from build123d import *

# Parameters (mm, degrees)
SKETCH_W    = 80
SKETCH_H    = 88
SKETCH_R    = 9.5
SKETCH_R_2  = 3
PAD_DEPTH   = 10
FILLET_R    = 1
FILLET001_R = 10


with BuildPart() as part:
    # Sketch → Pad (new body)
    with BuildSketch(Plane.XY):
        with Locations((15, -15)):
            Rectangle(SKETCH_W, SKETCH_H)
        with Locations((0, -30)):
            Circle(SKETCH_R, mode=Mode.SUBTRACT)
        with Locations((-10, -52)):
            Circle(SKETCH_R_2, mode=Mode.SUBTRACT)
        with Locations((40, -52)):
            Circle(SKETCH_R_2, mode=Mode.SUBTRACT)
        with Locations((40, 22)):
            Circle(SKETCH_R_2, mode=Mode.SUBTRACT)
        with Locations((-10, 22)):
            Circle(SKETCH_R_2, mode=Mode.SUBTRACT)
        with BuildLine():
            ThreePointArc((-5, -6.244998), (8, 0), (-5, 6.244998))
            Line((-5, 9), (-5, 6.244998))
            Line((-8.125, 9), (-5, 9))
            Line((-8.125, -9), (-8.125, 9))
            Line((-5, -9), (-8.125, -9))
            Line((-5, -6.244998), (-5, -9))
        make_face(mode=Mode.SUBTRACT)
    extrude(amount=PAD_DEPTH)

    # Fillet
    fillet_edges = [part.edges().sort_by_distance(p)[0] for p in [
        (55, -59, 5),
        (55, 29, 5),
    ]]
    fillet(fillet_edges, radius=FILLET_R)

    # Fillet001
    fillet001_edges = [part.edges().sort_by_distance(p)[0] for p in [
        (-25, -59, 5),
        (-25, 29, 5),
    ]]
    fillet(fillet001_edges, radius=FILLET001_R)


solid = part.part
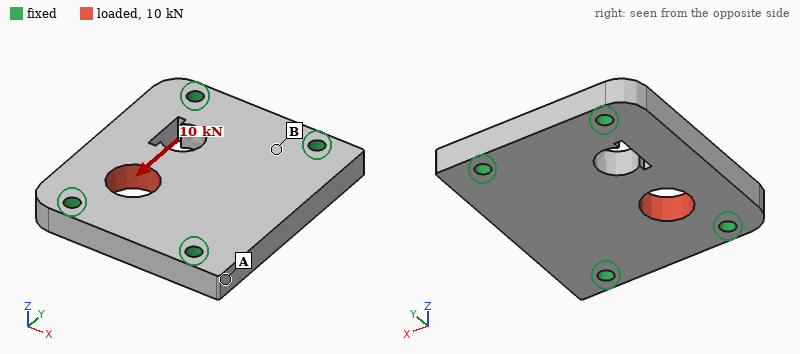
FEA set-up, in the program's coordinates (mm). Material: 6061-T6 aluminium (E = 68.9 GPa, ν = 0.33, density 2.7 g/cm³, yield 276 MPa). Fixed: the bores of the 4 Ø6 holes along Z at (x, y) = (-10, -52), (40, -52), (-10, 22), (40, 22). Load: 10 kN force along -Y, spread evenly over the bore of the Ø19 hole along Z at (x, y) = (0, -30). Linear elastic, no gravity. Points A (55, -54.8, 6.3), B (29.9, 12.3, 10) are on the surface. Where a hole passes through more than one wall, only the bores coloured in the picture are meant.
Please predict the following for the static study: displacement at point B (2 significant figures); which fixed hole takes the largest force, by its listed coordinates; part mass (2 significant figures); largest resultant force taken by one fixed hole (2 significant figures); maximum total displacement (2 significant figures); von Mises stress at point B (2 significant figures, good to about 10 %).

2.1 µm
(-10, -52)
170 g
4.8 kN
11 µm
9.9 MPa
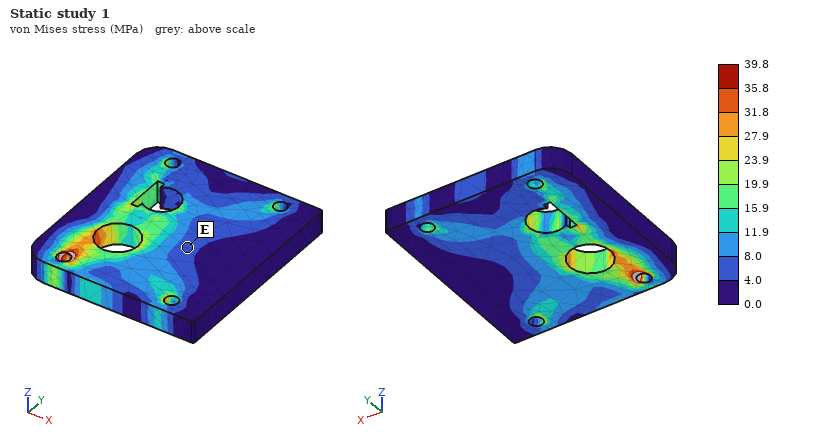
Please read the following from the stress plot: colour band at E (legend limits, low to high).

4.0 to 8.0 MPa
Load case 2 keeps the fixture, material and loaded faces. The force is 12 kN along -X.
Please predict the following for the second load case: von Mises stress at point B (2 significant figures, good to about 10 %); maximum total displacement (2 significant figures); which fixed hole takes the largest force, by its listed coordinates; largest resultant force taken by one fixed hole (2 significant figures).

13 MPa
21 µm
(-10, -52)
5.0 kN
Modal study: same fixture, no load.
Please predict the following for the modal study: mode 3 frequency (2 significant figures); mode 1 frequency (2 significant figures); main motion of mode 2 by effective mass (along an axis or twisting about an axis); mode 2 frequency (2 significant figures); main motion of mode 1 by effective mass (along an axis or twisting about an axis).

12 kHz
7300 Hz
twisting about Y
8900 Hz
along Z
